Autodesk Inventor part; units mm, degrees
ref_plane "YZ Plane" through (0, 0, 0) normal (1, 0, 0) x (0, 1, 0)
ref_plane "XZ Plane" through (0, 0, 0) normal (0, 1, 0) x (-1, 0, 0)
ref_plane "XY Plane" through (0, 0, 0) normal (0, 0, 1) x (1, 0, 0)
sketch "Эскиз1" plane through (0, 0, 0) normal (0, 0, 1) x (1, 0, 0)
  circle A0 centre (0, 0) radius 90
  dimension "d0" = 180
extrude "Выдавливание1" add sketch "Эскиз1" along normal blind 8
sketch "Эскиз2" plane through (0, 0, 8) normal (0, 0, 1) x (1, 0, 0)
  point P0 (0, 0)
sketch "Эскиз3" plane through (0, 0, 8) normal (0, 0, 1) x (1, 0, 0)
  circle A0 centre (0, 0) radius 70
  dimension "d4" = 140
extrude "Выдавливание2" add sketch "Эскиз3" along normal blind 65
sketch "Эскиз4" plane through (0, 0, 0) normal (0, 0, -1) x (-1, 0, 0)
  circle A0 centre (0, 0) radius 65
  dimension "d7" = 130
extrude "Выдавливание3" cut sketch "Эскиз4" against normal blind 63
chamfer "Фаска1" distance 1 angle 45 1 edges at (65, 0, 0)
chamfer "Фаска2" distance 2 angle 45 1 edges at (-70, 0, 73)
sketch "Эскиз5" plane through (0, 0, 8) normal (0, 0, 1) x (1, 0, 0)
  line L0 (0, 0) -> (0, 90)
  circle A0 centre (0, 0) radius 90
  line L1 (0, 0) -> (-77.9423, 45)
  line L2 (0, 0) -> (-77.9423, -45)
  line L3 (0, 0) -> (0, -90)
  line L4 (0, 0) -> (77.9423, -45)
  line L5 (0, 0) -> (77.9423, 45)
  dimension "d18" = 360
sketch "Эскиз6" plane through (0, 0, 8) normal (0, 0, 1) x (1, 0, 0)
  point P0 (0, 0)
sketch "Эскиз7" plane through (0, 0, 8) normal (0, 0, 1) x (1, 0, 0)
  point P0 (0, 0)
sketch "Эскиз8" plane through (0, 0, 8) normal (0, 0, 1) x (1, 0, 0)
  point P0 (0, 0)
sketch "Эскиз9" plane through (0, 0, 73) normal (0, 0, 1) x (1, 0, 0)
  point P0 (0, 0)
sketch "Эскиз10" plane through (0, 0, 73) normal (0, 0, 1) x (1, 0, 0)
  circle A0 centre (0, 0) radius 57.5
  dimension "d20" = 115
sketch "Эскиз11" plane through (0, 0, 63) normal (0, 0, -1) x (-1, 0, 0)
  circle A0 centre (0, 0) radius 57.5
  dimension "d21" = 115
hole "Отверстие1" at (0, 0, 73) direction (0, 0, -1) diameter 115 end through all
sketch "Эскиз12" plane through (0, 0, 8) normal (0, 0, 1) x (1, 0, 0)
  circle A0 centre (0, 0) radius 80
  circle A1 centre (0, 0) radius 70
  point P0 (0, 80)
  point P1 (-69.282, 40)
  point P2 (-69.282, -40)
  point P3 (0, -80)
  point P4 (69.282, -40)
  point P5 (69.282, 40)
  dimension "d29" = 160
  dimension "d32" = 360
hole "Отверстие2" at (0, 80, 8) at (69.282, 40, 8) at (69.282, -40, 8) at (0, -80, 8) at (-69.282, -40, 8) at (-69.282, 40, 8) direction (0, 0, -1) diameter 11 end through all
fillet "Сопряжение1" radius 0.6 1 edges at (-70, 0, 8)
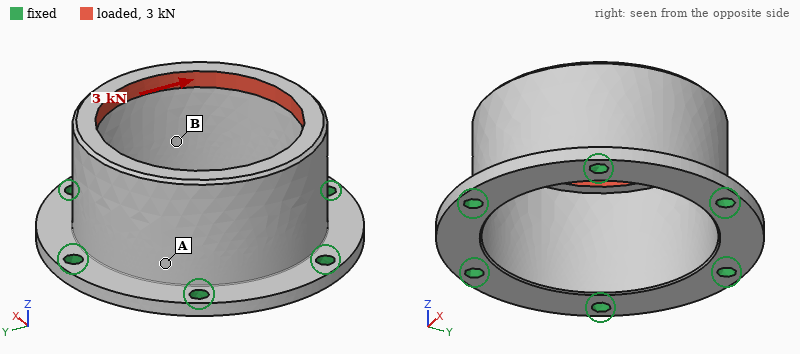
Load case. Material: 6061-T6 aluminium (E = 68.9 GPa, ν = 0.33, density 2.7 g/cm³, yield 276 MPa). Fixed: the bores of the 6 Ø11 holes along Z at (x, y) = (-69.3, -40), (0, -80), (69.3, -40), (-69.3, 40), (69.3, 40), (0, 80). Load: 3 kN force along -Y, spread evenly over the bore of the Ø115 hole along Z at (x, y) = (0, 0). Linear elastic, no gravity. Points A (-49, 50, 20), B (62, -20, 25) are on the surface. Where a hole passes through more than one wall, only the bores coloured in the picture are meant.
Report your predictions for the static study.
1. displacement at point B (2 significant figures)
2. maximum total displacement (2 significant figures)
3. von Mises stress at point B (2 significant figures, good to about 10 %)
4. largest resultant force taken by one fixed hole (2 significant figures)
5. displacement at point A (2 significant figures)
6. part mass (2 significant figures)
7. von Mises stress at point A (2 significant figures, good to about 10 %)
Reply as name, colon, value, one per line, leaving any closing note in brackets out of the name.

displacement at point B: 3.5 µm
maximum total displacement: 17 µm
von Mises stress at point B: 5.4 MPa
largest resultant force taken by one fixed hole: 950 N
displacement at point A: 4.2 µm
part mass: 700 g
von Mises stress at point A: 2.4 MPa
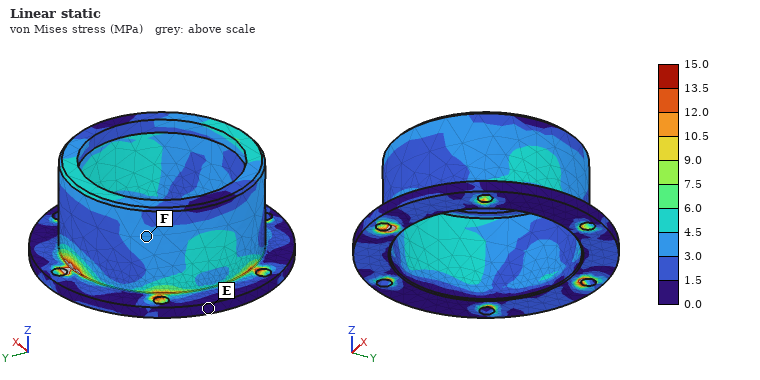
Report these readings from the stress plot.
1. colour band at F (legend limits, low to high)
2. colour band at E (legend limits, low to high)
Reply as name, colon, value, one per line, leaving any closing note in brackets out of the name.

colour band at F: 3.0 to 4.5 MPa
colour band at E: 0.0 to 1.5 MPa
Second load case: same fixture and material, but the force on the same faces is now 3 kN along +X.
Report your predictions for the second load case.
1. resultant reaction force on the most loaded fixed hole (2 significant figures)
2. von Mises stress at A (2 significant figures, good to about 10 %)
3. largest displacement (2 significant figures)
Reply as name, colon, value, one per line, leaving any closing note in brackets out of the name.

resultant reaction force on the most loaded fixed hole: 880 N
von Mises stress at A: 4.7 MPa
largest displacement: 17 µm
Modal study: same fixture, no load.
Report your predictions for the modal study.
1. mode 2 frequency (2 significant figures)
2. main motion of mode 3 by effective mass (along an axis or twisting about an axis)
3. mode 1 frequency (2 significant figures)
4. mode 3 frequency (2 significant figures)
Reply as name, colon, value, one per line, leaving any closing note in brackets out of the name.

mode 2 frequency: 3000 Hz
main motion of mode 3 by effective mass: along Y
mode 1 frequency: 3000 Hz
mode 3 frequency: 4700 Hz
